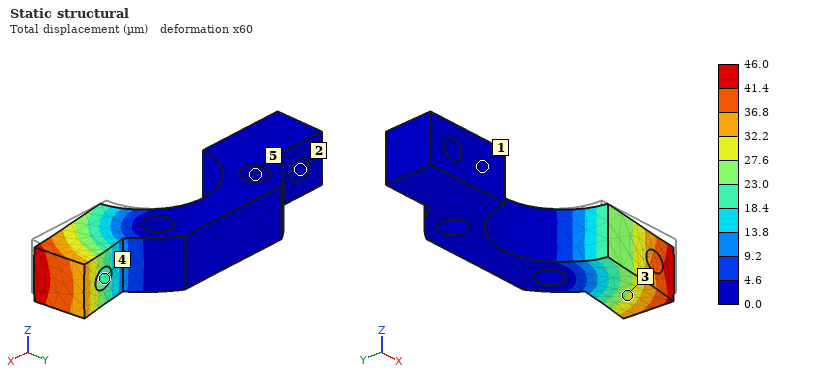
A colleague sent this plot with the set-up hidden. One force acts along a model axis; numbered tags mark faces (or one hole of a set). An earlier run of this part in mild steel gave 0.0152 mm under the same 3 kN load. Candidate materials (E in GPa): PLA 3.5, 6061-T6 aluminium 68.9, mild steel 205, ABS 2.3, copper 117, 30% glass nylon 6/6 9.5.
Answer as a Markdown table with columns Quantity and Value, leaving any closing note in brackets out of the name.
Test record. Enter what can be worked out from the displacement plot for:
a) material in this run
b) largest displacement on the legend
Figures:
| Quantity | Value |
|---|---|
| material in this run | 6061-T6 aluminium |
| largest displacement on the legend | 46.0 µm |
